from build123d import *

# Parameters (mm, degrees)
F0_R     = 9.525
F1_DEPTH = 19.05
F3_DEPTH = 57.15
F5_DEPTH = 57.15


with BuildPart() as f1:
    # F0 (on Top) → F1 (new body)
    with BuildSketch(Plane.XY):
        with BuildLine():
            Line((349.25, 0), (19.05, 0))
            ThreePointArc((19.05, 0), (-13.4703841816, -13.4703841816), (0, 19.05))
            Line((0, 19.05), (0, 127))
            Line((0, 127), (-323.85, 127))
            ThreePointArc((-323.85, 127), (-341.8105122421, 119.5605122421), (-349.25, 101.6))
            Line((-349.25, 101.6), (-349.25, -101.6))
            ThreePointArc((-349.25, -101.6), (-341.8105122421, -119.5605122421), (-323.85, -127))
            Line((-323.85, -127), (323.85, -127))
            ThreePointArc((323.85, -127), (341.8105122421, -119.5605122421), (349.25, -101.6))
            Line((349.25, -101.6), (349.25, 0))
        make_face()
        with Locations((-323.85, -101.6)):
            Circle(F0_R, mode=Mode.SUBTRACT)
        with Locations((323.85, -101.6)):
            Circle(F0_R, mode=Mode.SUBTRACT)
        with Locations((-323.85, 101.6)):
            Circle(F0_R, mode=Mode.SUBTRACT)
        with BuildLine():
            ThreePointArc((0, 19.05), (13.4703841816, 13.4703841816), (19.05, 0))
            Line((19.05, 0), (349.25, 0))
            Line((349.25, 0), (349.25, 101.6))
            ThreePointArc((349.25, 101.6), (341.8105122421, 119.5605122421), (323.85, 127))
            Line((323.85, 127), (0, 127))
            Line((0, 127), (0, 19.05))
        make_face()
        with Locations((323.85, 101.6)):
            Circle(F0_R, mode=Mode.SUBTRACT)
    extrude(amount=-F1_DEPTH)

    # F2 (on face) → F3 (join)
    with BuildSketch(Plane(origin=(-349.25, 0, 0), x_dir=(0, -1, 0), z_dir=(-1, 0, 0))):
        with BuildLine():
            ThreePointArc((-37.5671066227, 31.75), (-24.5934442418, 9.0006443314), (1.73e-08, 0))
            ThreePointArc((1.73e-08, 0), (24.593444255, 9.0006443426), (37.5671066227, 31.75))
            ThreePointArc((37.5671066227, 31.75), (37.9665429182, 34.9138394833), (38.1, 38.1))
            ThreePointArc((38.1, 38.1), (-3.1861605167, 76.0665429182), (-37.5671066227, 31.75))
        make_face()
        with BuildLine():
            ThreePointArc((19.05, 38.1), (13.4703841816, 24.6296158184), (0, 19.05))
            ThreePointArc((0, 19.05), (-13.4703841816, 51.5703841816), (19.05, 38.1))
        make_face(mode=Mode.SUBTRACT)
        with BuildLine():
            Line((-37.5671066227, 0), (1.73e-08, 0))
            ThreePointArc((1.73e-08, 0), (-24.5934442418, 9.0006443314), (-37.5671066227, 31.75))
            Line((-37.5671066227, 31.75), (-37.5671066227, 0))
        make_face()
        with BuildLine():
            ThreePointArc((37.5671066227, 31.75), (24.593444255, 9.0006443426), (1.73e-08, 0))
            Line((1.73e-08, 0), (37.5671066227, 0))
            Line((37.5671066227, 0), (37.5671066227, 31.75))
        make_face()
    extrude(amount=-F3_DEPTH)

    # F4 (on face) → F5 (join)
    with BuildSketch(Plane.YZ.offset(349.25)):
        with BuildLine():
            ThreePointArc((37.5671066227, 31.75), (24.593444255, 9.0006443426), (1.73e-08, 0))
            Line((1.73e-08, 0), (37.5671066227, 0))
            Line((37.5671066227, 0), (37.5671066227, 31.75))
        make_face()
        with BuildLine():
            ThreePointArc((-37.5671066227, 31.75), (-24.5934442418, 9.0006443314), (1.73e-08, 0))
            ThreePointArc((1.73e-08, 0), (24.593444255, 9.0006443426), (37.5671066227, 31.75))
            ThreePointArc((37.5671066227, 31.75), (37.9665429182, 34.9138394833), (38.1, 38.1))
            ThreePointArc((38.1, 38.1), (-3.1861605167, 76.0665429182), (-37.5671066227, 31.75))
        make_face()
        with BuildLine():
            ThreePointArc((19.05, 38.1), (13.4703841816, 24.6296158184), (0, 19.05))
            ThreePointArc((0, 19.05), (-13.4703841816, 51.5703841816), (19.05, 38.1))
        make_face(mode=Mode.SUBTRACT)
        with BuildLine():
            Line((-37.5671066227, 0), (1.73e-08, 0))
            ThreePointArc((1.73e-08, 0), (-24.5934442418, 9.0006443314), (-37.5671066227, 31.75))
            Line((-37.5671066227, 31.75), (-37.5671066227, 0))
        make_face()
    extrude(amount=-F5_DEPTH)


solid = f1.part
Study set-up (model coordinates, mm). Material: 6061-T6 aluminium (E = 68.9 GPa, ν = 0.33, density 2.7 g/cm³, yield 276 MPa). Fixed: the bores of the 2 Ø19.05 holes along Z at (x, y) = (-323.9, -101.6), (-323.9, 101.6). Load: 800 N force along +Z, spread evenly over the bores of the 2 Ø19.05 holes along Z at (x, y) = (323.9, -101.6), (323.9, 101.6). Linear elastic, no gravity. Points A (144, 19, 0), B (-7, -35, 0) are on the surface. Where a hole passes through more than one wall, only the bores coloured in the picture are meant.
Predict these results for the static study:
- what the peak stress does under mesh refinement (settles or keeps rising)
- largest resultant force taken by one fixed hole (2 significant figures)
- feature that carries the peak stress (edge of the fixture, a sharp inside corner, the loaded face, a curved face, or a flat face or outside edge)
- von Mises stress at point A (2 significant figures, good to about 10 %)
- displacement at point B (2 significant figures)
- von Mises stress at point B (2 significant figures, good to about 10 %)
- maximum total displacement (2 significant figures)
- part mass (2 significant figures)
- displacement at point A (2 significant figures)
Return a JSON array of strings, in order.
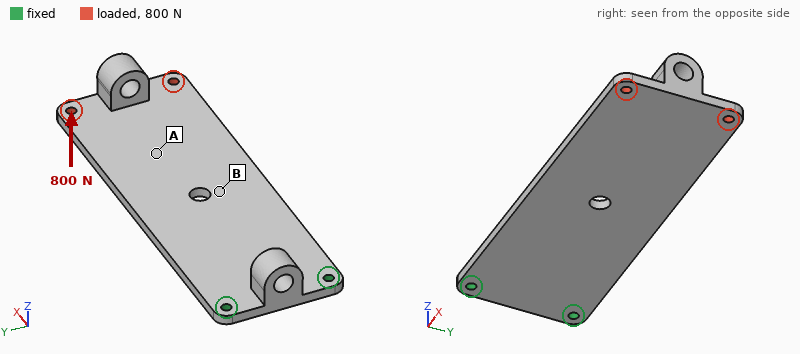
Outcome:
["keeps rising", "400 N", "edge of the fixture", "9.3 MPa", "2.4 mm", "22 MPa", "8.3 mm", "10 kg", "4.7 mm"]
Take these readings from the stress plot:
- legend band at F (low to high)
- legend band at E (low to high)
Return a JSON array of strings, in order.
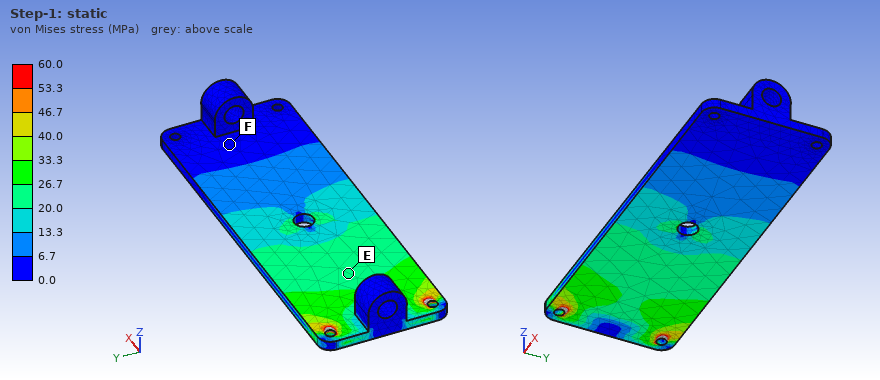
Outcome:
["0.0 to 6.7 MPa", "20.0 to 26.7 MPa"]
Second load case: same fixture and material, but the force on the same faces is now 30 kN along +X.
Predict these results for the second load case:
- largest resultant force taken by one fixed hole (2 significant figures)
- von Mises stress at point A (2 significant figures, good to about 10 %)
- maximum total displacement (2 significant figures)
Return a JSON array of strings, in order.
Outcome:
["15 kN", "5.2 MPa", "82 µm"]
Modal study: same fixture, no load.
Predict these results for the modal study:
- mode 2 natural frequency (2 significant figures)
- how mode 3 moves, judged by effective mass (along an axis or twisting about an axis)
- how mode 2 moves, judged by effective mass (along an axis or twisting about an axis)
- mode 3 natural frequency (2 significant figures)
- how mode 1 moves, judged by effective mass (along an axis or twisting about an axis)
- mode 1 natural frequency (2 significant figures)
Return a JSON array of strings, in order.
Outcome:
["180 Hz", "along Z", "twisting about X", "190 Hz", "along Z", "30 Hz"]
